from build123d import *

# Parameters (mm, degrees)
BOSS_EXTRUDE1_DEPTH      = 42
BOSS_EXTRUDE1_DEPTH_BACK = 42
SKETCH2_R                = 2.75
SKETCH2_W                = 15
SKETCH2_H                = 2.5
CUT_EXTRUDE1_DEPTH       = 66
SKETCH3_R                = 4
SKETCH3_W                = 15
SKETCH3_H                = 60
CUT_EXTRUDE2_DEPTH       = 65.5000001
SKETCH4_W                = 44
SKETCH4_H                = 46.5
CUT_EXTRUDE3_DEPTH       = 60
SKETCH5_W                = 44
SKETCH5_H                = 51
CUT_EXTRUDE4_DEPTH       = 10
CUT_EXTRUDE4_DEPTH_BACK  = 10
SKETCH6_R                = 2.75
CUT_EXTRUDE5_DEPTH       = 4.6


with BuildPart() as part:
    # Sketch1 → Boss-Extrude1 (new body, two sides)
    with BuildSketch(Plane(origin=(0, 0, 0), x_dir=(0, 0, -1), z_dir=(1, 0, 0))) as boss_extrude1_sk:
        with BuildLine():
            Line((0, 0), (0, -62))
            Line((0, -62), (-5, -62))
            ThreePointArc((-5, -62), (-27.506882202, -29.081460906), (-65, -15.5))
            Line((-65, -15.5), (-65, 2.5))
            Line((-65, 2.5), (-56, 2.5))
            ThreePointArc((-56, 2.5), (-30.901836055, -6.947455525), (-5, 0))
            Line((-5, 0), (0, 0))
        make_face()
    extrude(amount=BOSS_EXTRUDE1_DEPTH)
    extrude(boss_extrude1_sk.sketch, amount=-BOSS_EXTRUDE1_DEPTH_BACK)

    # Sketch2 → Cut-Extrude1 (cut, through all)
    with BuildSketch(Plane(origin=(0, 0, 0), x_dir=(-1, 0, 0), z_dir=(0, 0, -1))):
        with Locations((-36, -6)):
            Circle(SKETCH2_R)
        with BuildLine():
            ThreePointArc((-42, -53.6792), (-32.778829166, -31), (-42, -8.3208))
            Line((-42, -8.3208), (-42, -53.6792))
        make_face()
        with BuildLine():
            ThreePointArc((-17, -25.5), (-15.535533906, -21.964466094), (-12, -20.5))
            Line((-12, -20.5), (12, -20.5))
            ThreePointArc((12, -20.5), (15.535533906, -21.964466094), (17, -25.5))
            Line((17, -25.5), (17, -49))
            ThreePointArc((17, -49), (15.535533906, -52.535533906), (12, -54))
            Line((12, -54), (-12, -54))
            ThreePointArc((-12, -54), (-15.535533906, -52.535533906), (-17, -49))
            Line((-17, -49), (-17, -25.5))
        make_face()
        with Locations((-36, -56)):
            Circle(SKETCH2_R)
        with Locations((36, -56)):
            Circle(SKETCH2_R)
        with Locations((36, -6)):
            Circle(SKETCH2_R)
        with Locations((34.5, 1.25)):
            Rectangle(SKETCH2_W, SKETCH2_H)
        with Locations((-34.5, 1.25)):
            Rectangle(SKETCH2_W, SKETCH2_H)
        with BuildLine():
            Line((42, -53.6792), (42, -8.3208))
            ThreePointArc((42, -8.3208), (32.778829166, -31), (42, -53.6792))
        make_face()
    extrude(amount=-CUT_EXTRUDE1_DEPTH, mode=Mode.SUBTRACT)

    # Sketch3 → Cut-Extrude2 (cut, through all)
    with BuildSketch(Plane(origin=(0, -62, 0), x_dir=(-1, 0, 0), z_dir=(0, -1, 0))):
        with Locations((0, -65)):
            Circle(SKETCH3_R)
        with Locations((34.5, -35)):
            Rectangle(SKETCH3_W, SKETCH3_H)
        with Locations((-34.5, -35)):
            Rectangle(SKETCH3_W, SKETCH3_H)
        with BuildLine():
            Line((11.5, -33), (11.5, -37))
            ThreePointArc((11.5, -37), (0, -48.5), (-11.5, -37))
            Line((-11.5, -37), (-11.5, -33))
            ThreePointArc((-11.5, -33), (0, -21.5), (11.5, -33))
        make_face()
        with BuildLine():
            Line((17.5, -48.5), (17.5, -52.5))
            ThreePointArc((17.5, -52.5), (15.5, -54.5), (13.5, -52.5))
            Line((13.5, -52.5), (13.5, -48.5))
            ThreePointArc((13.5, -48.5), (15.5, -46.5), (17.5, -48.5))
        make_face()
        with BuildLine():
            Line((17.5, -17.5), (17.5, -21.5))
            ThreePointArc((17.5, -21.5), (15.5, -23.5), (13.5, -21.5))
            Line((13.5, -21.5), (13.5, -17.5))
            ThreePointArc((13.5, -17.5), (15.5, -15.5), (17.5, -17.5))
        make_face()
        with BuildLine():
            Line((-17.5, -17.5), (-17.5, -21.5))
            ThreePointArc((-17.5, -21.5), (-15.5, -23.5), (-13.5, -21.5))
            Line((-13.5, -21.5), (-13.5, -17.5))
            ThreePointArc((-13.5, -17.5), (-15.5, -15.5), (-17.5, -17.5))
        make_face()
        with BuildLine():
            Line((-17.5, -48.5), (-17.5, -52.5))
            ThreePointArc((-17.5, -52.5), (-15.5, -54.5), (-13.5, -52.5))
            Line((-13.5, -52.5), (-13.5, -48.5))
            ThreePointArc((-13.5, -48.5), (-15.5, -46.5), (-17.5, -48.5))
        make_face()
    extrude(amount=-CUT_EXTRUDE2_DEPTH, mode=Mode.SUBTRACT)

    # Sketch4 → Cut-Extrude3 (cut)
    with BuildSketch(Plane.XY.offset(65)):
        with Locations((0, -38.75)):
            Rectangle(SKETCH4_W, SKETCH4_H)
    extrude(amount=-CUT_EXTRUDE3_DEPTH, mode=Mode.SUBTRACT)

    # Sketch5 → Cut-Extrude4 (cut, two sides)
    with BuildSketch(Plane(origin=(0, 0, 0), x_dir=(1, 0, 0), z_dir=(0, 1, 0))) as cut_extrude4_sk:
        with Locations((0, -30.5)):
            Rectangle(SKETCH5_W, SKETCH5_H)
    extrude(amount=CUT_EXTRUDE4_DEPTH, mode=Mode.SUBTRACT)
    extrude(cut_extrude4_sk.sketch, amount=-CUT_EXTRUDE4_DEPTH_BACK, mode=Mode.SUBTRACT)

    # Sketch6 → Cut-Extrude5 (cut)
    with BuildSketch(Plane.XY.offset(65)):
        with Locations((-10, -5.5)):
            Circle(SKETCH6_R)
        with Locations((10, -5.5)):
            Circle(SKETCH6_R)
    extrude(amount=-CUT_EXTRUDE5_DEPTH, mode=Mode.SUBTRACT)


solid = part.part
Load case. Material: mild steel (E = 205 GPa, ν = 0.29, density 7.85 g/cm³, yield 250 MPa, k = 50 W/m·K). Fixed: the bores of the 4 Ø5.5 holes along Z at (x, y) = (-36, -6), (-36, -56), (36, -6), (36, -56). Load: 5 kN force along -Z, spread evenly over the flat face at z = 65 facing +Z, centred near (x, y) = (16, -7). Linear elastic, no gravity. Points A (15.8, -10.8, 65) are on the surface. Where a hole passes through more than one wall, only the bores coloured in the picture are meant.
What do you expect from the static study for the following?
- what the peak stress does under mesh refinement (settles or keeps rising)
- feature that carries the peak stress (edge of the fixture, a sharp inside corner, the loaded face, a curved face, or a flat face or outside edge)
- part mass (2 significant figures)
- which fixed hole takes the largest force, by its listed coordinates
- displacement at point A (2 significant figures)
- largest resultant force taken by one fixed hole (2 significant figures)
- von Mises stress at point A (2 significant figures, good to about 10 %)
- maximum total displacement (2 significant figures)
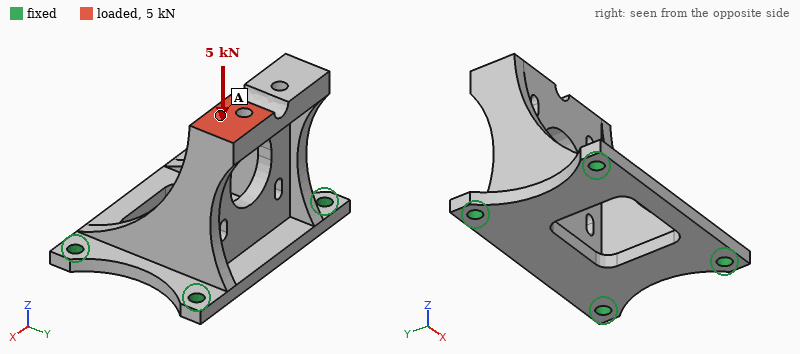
keeps rising
edge of the fixture
370 g
(36, -6)
0.080 mm
3.8 kN
22 MPa
0.10 mm
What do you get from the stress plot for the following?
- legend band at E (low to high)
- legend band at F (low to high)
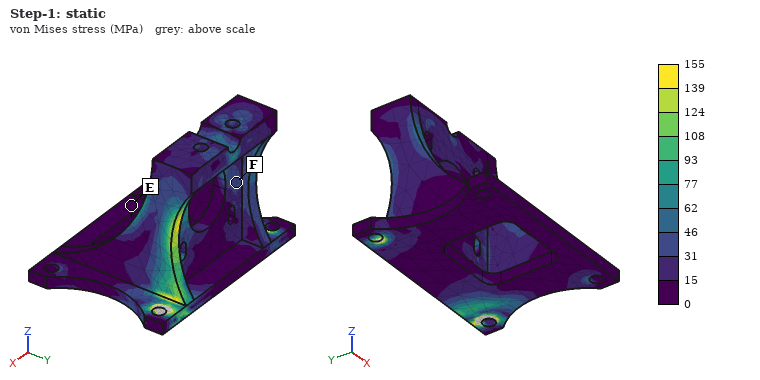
0 to 15 MPa
31 to 46 MPa
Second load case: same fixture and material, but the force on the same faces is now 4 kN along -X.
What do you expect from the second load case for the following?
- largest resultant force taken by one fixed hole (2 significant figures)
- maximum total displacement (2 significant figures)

3.6 kN
73 µm
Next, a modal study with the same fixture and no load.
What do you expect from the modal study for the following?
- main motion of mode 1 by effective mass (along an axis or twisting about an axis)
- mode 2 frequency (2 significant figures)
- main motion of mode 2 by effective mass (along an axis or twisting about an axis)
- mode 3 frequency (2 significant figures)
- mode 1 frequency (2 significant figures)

along Y
3900 Hz
along X
4500 Hz
2500 Hz
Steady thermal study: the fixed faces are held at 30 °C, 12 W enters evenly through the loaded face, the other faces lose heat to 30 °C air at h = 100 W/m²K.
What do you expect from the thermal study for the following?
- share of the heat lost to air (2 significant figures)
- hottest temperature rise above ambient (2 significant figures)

87 %
27 K
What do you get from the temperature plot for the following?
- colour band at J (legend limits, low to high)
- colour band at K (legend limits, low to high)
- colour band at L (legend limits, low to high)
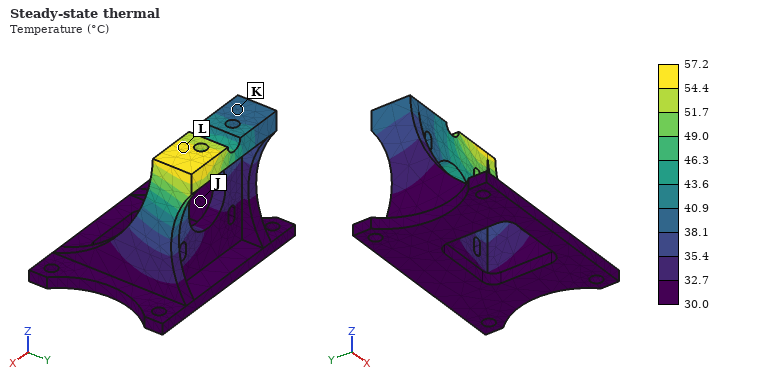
30.0 to 32.7 °C
38.1 to 40.9 °C
54.4 to 57.2 °C
